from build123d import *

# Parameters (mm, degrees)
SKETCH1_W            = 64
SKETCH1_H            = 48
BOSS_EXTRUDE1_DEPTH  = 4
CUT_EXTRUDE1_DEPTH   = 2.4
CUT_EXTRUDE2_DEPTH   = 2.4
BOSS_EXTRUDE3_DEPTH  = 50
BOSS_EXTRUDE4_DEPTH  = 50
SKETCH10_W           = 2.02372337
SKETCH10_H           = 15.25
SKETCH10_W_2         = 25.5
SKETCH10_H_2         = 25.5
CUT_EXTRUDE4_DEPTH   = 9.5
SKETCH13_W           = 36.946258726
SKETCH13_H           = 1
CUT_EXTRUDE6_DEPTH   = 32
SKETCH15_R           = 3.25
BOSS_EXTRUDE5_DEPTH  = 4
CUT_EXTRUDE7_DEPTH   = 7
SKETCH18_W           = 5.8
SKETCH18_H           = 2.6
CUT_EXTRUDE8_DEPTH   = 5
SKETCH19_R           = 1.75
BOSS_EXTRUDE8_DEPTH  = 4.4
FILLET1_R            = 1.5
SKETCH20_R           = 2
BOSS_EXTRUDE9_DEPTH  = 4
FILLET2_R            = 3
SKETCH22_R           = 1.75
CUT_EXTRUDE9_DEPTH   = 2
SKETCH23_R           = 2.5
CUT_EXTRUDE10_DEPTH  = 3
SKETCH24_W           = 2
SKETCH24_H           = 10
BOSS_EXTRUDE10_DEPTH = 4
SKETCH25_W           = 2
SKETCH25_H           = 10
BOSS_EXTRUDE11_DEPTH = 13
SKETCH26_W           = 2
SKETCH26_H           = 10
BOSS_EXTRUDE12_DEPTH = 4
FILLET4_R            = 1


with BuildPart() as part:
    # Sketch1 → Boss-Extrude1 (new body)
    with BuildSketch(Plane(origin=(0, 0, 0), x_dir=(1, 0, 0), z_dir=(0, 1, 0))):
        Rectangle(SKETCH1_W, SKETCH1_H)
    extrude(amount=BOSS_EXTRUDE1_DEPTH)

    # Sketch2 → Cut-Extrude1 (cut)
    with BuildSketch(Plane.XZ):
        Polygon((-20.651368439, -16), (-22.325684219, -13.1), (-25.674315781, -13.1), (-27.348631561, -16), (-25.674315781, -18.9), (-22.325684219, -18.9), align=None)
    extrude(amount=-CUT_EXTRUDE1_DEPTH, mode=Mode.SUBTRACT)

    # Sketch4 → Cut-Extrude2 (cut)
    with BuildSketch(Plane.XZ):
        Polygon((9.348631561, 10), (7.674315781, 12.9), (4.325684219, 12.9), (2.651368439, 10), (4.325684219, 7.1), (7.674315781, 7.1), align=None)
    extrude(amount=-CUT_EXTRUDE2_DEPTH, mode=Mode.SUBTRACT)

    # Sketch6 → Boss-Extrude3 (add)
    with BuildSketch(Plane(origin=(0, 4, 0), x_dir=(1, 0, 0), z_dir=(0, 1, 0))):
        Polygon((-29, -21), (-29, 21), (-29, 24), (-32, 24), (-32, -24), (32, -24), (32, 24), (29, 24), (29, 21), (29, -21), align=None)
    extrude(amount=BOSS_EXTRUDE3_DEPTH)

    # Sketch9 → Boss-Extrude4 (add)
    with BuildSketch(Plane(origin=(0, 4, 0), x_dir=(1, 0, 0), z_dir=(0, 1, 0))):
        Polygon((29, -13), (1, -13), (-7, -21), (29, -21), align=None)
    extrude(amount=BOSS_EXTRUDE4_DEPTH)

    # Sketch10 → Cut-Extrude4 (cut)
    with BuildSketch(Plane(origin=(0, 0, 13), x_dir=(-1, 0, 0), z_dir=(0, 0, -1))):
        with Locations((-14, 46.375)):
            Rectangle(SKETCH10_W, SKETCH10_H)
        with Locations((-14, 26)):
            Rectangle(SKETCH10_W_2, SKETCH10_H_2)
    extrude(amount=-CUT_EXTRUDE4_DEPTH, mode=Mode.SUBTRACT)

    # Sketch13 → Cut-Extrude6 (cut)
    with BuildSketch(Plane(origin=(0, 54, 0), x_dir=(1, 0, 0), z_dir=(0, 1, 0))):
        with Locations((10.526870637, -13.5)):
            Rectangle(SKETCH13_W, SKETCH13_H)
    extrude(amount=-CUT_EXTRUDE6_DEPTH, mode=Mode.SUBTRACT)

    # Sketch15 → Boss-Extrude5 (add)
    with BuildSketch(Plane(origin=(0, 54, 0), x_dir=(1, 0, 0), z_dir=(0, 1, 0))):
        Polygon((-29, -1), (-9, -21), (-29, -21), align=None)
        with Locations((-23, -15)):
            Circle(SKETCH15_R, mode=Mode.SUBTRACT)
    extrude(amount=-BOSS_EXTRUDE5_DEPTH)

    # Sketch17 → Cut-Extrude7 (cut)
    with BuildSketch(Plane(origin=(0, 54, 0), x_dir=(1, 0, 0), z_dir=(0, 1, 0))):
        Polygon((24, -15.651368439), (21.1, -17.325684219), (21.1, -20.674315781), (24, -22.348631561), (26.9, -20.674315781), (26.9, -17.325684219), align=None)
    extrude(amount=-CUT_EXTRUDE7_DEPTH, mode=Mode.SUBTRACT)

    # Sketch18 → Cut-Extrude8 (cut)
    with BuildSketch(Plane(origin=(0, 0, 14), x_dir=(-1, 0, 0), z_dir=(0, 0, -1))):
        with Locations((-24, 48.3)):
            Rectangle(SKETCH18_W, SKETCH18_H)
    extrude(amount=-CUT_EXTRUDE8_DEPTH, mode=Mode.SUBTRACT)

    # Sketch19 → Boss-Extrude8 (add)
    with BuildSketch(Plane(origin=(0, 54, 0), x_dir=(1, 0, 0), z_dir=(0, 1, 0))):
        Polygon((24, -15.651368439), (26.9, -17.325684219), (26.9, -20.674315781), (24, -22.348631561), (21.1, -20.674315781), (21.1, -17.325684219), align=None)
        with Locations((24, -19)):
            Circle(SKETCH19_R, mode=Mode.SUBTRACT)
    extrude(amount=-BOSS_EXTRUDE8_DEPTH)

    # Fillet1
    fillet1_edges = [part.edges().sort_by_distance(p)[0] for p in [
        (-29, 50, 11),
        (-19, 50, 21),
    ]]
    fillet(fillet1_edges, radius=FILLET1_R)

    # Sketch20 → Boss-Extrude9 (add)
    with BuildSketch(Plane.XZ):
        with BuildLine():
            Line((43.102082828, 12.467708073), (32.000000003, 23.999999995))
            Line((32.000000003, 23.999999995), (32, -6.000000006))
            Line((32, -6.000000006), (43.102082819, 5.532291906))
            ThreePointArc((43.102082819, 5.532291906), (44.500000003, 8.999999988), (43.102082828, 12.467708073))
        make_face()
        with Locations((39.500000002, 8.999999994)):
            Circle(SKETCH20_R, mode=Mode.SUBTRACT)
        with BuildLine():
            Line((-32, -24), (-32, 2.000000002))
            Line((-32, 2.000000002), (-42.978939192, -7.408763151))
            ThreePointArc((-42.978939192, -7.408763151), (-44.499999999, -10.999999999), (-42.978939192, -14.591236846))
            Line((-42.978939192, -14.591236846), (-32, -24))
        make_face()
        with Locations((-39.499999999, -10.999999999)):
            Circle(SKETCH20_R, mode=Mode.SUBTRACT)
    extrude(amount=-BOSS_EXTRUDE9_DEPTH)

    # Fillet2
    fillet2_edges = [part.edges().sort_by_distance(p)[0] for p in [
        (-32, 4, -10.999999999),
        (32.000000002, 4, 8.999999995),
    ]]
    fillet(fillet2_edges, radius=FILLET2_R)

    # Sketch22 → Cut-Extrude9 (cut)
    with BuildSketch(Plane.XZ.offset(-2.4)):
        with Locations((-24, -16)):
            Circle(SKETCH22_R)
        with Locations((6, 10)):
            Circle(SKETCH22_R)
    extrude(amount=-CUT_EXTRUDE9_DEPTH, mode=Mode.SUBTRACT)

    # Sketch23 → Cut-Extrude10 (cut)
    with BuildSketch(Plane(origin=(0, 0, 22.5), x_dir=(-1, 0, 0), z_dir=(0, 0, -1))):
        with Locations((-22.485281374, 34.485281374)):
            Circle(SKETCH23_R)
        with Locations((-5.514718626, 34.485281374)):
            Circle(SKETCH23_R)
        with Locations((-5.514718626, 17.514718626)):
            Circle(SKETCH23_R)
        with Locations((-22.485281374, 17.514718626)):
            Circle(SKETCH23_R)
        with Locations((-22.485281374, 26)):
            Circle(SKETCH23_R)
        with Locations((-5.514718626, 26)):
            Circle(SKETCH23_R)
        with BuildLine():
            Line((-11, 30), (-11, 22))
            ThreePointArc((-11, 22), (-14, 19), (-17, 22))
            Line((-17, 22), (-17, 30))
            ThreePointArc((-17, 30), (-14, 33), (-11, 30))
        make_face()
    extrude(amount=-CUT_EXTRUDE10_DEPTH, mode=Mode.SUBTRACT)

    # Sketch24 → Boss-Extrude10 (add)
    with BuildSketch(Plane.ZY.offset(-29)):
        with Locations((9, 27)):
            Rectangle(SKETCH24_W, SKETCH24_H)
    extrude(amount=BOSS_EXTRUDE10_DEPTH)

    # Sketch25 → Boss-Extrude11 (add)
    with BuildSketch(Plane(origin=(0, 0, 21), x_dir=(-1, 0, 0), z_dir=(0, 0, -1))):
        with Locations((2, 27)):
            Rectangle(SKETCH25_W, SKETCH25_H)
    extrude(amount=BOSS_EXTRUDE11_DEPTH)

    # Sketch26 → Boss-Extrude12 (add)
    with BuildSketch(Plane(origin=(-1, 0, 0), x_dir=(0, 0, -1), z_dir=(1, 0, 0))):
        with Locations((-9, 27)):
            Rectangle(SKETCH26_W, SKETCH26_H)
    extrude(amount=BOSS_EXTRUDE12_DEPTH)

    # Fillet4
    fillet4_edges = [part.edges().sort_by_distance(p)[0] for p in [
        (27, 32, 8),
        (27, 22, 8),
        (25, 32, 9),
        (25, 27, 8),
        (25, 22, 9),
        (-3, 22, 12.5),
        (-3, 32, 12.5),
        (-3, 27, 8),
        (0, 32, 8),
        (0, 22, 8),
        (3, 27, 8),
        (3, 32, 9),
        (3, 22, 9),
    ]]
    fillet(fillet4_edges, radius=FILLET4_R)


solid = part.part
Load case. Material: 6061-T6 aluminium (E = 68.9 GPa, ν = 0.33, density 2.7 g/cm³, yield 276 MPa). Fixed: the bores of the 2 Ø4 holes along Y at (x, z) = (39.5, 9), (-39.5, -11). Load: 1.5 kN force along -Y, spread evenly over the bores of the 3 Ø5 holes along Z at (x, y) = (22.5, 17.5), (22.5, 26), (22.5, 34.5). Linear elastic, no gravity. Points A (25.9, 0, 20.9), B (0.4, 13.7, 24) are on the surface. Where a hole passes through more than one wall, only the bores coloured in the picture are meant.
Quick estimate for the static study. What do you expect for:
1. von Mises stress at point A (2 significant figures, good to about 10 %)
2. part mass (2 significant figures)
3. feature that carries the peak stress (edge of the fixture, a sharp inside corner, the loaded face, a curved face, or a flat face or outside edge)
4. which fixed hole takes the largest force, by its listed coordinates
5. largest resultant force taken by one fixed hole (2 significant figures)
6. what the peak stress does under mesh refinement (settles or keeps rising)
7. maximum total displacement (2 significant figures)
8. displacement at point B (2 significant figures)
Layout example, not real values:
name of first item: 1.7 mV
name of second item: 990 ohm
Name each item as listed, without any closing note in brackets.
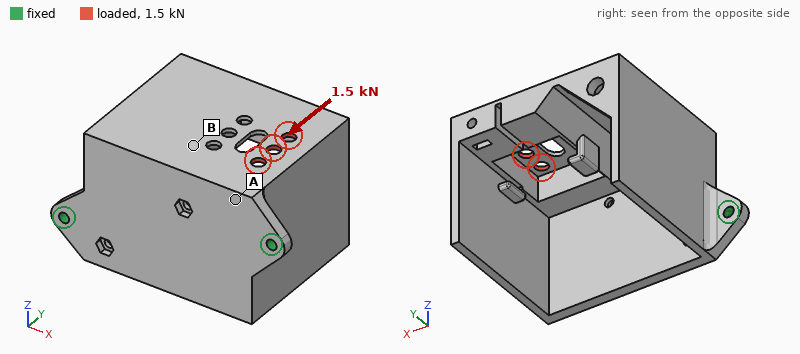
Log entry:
von Mises stress at point A: 32 MPa
part mass: 120 g
feature that carries the peak stress: edge of the fixture
which fixed hole takes the largest force, by its listed coordinates: (39.5, 9)
largest resultant force taken by one fixed hole: 1.3 kN
what the peak stress does under mesh refinement: keeps rising
maximum total displacement: 0.56 mm
displacement at point B: 0.25 mm
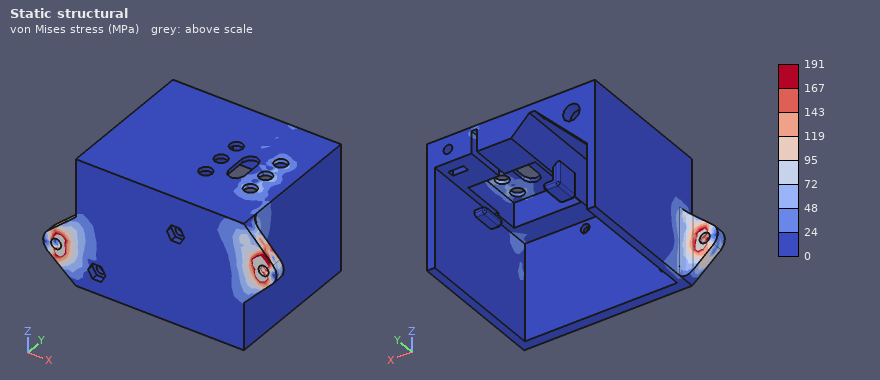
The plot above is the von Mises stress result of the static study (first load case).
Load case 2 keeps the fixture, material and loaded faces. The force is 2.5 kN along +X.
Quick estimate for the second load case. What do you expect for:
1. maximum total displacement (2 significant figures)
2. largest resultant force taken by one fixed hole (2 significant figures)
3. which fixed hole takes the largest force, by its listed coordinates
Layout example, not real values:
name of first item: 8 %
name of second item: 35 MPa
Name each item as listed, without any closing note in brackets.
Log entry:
maximum total displacement: 0.58 mm
largest resultant force taken by one fixed hole: 2.0 kN
which fixed hole takes the largest force, by its listed coordinates: (39.5, 9)
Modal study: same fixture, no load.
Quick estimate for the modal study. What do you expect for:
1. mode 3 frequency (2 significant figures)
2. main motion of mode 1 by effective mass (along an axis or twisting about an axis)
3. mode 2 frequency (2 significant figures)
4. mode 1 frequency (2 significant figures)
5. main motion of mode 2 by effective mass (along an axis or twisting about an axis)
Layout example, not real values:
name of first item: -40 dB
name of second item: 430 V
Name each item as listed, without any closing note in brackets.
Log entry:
mode 3 frequency: 1900 Hz
main motion of mode 1 by effective mass: along Z
mode 2 frequency: 1400 Hz
mode 1 frequency: 790 Hz
main motion of mode 2 by effective mass: along X
